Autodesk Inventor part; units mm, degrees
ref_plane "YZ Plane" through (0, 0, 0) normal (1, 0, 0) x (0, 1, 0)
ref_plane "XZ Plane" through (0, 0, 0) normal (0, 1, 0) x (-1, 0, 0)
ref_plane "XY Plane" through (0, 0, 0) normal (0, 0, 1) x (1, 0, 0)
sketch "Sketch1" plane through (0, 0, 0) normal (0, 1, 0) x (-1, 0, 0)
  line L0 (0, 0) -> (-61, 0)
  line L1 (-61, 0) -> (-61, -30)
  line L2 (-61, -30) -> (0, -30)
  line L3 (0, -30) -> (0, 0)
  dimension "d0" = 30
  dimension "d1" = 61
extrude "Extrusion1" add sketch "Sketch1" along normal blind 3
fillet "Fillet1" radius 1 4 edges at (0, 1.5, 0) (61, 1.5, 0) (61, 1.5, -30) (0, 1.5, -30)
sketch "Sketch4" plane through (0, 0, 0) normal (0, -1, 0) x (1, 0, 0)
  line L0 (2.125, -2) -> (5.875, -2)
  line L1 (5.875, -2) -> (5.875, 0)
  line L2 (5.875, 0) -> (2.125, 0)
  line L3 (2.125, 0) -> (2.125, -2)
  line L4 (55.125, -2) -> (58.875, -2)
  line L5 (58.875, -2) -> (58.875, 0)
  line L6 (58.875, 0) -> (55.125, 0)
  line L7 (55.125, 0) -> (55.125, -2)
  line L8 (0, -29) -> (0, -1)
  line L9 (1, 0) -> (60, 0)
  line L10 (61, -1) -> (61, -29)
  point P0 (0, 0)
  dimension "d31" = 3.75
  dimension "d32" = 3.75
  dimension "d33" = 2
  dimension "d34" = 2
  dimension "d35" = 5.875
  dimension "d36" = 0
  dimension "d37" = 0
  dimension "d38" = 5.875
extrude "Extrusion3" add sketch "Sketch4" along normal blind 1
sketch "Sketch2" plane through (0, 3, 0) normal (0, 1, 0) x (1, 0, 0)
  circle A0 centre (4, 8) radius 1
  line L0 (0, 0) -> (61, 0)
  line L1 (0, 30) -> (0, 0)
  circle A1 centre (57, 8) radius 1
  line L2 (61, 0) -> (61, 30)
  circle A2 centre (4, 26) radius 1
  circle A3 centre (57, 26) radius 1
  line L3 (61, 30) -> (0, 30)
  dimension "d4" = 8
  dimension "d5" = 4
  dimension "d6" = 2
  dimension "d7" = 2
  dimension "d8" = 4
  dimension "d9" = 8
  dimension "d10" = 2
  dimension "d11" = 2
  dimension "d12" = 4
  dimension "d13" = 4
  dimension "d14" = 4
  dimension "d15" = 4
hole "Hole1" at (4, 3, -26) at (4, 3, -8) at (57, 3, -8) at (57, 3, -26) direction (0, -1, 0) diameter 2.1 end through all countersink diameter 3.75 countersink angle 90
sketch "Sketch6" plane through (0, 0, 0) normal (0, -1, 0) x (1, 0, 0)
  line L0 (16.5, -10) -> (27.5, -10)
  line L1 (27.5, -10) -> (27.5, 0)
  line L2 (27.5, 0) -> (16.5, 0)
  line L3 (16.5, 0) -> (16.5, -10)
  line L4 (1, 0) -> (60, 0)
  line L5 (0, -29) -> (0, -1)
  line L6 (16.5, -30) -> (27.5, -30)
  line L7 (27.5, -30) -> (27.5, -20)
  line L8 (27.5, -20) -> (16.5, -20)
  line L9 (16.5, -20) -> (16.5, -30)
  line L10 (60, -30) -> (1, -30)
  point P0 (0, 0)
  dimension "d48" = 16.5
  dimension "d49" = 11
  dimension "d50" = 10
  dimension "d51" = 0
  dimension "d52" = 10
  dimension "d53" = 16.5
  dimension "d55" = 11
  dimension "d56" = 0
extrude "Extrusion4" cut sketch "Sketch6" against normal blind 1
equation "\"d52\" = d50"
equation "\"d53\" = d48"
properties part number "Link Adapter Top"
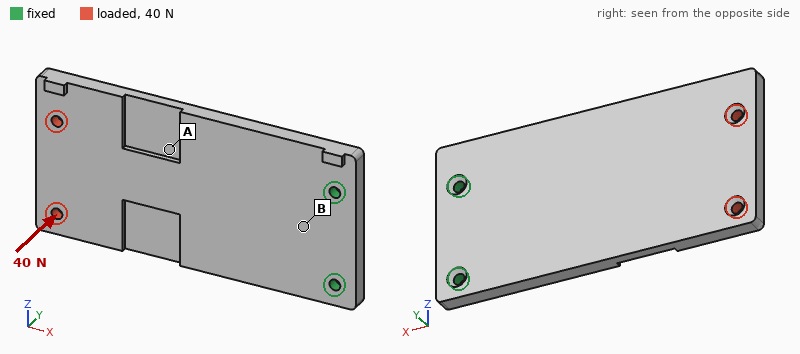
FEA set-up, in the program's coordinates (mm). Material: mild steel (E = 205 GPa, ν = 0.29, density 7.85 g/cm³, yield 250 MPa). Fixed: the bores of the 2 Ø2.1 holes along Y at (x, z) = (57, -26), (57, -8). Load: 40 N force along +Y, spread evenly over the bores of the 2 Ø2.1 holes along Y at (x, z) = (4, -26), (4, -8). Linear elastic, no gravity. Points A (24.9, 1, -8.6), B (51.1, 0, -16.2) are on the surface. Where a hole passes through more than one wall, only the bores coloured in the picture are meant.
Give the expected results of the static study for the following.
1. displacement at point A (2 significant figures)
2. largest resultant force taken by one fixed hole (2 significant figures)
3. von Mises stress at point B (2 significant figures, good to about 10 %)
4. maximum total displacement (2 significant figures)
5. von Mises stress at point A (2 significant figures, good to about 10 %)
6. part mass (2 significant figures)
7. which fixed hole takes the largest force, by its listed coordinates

0.076 mm
24 N
37 MPa
0.20 mm
18 MPa
41 g
(57, -8)
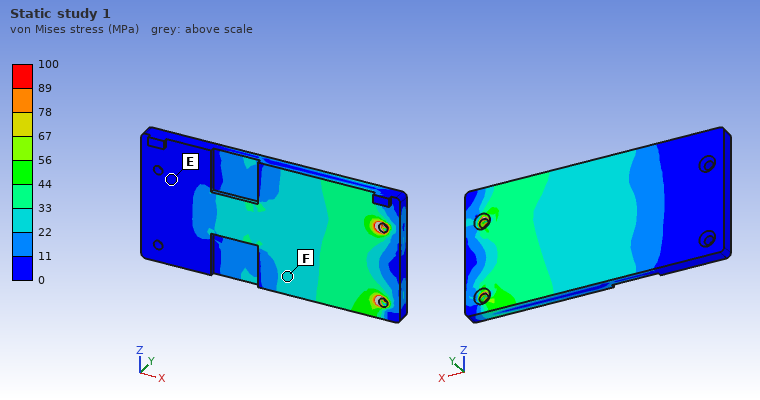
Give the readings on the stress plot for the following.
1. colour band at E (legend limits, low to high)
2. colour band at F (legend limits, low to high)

0 to 11 MPa
22 to 33 MPa
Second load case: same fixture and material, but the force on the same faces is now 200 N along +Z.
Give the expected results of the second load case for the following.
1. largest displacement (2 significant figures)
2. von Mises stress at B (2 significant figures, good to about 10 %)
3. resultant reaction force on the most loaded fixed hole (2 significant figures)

16 µm
11 MPa
580 N
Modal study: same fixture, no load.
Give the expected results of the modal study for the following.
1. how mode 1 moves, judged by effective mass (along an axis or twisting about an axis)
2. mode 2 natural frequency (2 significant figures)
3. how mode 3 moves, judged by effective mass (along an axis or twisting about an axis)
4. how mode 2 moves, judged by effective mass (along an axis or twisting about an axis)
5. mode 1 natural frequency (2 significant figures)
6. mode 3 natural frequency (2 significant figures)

along Y
2900 Hz
along Y
twisting about X
710 Hz
4000 Hz
